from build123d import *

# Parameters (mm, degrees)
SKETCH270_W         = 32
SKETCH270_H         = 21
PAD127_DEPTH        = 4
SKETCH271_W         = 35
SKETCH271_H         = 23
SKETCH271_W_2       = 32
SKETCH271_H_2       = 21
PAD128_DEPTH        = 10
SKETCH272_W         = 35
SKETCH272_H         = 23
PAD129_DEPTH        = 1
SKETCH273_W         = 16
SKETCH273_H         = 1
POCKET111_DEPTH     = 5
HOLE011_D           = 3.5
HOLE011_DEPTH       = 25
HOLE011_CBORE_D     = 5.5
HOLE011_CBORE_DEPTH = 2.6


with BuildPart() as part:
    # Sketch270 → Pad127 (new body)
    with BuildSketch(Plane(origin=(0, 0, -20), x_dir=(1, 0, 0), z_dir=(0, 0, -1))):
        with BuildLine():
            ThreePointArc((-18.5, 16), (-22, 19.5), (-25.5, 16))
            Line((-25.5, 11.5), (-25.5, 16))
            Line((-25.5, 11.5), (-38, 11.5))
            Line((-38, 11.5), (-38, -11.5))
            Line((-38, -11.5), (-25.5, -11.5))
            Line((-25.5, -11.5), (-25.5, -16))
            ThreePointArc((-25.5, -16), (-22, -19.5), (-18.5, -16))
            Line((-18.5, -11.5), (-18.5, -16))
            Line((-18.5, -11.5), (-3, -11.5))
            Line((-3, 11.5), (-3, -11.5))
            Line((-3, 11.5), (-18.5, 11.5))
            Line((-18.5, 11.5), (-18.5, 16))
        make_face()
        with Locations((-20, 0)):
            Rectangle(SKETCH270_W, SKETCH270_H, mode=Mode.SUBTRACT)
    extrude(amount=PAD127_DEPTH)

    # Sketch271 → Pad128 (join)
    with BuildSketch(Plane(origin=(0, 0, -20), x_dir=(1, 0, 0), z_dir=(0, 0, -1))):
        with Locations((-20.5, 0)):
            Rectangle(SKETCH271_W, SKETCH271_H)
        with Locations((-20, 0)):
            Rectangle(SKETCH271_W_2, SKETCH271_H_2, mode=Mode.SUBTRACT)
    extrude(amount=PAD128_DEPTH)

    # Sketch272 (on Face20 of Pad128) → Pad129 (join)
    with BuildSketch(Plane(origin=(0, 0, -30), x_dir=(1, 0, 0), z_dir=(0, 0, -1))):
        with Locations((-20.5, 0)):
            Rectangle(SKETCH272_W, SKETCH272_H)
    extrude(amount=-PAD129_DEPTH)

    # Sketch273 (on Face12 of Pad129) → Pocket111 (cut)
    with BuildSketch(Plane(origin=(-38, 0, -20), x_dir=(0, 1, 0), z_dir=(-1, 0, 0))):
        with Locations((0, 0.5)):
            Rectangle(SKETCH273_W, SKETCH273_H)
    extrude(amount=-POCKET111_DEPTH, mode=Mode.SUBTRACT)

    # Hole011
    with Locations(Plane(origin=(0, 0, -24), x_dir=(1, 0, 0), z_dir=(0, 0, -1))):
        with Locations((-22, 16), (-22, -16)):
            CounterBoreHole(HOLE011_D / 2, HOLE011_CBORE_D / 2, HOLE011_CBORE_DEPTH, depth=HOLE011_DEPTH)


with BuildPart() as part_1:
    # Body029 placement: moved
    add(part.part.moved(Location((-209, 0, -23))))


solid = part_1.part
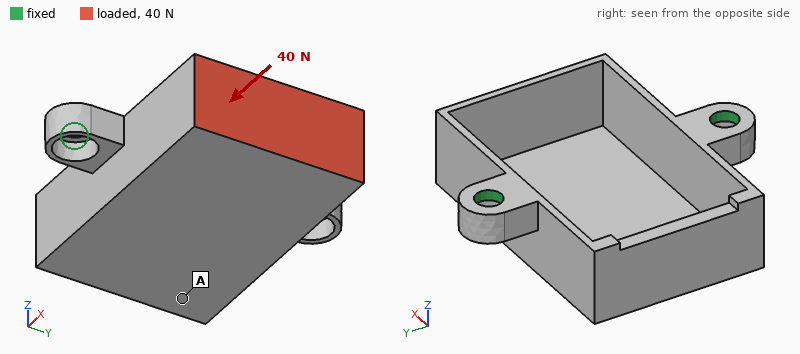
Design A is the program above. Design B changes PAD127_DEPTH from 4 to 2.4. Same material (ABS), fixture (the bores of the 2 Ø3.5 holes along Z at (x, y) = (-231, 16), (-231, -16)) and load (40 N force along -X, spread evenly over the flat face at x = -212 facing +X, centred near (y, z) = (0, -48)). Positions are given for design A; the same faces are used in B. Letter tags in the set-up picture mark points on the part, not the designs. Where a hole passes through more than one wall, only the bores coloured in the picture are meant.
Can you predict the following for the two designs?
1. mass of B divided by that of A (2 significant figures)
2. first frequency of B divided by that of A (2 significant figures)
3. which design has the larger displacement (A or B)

0.96
0.73
B
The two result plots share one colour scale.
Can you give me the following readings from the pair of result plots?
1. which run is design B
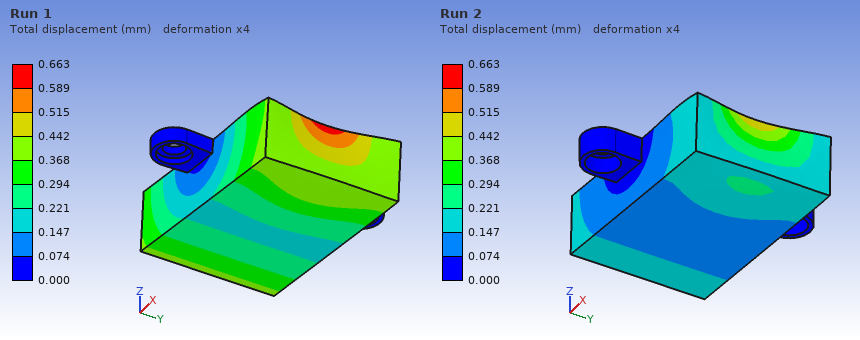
Run 1
